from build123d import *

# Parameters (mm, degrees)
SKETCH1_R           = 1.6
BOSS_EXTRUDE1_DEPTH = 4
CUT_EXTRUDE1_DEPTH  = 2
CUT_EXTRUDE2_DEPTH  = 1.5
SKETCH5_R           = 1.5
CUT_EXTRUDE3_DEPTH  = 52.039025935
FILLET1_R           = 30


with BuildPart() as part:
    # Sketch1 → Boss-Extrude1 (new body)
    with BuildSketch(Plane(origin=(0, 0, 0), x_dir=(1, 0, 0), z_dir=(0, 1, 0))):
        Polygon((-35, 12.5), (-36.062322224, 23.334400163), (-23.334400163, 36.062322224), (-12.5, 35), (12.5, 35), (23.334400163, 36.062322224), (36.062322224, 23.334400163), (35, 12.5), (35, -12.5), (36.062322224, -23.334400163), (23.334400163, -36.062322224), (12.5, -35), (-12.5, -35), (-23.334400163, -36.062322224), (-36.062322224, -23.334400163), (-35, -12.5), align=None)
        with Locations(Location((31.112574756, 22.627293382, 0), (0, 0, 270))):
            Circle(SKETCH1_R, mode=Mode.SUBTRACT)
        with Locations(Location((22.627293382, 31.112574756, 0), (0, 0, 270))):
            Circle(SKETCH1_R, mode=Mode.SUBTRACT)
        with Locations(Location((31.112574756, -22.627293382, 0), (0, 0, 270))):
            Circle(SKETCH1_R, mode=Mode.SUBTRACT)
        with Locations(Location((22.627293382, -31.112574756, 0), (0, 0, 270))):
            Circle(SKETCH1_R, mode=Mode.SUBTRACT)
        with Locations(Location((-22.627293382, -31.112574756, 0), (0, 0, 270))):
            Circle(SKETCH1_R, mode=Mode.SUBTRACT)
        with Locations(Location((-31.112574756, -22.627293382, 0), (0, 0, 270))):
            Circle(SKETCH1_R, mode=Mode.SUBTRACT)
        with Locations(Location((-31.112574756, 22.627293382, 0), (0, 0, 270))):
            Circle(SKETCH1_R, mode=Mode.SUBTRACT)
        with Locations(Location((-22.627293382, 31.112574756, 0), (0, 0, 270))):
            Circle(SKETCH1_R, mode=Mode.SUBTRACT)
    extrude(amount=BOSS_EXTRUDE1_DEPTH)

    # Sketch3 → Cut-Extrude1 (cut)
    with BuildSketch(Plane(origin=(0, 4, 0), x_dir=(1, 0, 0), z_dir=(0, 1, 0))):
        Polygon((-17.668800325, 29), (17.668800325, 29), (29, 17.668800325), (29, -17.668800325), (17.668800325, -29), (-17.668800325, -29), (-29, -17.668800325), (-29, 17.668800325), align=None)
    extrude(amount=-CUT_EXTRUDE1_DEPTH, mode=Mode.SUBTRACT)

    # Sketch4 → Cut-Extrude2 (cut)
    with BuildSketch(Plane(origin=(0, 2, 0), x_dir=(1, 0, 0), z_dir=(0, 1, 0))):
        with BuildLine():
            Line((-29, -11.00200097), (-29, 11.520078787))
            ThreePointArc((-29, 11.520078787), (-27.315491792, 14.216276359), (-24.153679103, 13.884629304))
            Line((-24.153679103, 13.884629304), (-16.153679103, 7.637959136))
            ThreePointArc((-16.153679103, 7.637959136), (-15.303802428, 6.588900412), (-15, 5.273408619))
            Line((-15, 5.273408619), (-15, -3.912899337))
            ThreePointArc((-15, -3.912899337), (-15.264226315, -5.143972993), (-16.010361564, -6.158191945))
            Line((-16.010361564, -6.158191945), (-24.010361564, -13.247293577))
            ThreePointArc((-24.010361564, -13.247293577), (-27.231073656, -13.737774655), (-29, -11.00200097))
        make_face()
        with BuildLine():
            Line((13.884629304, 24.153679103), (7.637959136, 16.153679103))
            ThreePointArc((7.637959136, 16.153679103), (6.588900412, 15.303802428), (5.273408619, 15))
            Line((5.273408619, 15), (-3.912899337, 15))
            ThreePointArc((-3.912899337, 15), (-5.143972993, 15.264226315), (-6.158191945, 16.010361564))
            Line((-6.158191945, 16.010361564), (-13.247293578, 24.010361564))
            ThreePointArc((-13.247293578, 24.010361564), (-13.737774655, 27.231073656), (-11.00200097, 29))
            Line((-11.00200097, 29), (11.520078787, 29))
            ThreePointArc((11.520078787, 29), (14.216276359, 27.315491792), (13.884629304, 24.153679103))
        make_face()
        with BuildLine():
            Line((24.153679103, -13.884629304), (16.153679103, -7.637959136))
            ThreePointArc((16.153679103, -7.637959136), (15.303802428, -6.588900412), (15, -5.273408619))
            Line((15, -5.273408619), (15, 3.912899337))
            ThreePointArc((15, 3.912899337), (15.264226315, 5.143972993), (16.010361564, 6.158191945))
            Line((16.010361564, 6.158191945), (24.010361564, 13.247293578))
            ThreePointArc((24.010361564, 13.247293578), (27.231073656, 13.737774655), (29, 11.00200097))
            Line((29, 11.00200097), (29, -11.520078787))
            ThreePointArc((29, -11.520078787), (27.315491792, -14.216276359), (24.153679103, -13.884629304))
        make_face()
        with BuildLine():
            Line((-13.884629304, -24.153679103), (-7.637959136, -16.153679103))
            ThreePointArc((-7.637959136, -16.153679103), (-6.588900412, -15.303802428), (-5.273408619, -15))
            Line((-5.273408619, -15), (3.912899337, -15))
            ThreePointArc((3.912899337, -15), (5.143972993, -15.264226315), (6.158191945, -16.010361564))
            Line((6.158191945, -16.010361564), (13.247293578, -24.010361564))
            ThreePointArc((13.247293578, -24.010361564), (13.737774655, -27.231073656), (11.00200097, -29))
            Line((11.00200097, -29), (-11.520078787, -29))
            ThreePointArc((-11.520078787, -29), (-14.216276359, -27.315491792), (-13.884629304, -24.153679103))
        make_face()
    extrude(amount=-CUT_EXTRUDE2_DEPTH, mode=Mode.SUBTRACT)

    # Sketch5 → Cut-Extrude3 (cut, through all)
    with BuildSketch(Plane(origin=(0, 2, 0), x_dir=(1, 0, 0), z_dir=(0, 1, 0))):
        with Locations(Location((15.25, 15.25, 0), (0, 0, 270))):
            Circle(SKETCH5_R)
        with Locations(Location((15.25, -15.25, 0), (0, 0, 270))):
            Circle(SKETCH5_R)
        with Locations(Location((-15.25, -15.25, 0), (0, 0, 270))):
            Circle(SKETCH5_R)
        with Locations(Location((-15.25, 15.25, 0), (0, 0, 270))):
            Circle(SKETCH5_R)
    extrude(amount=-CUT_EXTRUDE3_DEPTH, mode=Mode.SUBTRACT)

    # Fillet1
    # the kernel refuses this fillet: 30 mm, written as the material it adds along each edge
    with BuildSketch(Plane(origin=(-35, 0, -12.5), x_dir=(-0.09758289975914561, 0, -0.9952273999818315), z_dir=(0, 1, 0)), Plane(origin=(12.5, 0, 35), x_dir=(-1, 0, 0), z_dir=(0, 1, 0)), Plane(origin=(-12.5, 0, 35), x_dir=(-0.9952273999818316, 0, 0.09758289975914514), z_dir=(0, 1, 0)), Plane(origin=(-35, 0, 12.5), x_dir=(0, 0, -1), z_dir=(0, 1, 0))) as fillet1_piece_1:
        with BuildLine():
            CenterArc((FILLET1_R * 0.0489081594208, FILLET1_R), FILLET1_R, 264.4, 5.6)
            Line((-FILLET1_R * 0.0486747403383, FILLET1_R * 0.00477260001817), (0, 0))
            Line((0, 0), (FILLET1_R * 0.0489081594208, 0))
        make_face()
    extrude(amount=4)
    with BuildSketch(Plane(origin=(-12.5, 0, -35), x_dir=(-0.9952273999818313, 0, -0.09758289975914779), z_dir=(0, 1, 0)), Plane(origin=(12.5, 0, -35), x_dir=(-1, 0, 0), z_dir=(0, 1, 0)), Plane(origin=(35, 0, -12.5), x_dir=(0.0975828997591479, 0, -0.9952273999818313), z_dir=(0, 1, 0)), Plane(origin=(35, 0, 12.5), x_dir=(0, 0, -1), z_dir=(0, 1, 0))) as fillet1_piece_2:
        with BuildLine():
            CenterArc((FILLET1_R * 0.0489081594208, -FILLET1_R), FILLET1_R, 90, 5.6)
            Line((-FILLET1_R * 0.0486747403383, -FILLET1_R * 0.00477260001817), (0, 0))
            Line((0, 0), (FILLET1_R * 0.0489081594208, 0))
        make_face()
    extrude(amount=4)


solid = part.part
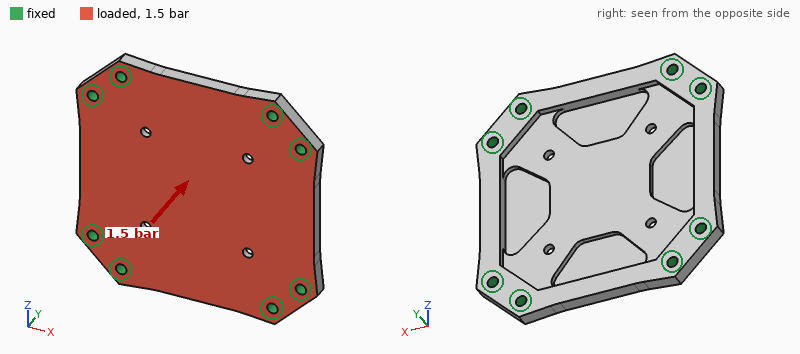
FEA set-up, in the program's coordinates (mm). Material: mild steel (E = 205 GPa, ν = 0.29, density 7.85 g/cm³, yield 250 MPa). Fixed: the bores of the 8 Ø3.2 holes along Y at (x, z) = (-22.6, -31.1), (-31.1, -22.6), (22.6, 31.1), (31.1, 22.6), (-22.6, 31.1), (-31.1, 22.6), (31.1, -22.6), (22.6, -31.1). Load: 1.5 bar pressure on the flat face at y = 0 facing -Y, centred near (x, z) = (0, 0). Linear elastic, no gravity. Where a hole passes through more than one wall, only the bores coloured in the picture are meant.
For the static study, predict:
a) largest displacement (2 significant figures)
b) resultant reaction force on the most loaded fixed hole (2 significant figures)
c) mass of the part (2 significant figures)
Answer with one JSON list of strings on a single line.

["39 µm", "110 N", "82 g"]
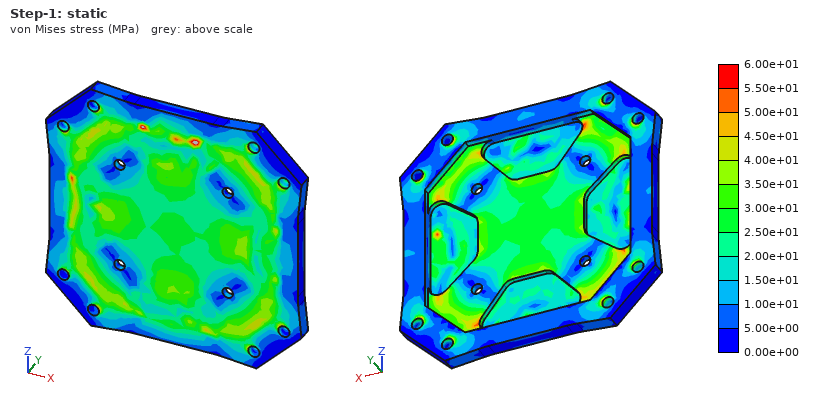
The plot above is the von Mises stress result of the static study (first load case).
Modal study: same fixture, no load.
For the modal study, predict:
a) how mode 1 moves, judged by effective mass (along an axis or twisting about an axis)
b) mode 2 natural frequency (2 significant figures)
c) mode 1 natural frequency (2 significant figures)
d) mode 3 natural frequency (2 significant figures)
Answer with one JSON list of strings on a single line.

["along Y", "6900 Hz", "3300 Hz", "7000 Hz"]
